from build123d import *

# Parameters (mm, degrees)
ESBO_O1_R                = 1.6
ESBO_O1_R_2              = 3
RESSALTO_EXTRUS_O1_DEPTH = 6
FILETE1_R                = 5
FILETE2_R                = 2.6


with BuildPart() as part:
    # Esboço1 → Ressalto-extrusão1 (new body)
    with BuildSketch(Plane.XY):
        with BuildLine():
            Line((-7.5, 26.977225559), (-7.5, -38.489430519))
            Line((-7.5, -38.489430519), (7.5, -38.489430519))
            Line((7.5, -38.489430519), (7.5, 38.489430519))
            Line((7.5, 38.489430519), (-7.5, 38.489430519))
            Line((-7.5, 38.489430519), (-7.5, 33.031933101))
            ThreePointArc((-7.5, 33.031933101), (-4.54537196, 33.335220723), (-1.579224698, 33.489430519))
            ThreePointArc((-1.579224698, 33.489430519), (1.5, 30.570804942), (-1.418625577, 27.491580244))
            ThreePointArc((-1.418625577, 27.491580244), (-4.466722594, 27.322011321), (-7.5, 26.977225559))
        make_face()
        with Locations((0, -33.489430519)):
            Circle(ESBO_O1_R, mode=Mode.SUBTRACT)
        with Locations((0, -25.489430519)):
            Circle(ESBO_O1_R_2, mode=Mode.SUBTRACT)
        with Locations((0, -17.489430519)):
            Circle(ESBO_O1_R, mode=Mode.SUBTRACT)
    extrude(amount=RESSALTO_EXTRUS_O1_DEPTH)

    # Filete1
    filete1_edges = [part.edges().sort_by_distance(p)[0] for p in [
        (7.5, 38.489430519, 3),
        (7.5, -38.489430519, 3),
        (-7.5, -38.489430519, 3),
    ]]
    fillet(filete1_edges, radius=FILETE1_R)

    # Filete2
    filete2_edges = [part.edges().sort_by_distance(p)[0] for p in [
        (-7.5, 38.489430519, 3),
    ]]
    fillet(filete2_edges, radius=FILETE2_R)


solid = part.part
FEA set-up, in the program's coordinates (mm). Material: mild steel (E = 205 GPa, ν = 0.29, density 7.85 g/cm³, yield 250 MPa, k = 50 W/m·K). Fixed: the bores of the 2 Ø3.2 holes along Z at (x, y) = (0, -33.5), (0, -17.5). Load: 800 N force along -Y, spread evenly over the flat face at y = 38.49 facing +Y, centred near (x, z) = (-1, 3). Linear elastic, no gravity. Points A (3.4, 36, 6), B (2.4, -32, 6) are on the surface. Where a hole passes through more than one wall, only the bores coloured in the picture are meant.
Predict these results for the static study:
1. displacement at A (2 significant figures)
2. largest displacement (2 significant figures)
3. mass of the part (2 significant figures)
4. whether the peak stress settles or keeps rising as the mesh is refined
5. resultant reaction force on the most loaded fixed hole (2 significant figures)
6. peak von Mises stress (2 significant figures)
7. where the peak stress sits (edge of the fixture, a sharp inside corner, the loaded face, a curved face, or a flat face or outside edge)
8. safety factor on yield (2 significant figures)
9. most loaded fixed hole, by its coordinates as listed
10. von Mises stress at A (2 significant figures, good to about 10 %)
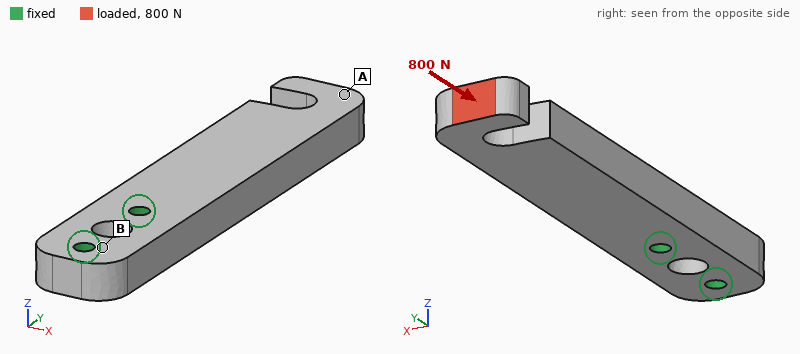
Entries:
15 µm
32 µm
49 g
settles
690 N
220 MPa
a curved face
1.2
(0, -17.5)
36 MPa
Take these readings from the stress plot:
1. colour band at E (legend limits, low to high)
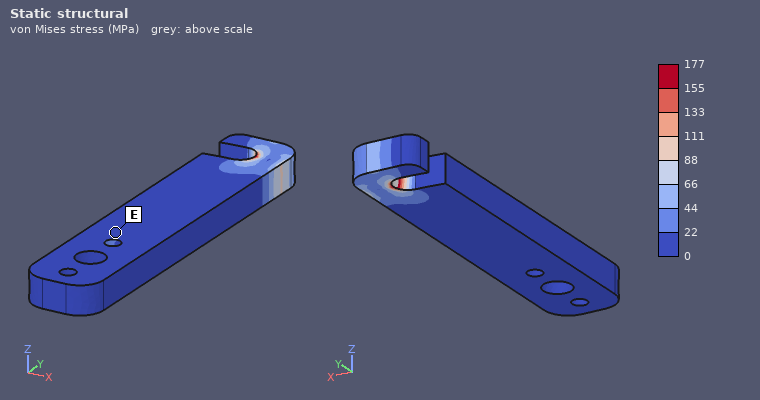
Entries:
0 to 22 MPa
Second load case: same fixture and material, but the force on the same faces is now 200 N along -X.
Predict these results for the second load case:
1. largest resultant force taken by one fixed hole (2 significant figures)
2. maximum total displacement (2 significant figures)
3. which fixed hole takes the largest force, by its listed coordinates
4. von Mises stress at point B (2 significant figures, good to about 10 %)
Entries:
600 N
57 µm
(0, -17.5)
16 MPa
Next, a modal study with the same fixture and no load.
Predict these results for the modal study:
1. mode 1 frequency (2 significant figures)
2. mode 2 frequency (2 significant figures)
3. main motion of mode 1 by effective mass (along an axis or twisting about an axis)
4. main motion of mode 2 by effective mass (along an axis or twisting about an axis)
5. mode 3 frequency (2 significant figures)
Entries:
1700 Hz
3400 Hz
along Z
along X
9000 Hz
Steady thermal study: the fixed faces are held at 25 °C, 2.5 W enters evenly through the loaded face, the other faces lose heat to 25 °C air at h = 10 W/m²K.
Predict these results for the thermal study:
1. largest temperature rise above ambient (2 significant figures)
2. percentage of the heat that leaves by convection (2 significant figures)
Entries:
41 K
15 %
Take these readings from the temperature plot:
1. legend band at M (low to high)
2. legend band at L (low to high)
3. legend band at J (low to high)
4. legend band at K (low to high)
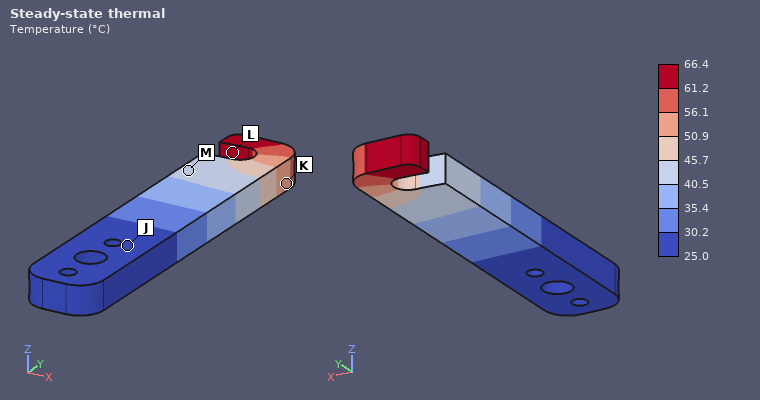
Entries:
40.5 to 45.7 °C
61.2 to 66.4 °C
25.0 to 30.2 °C
50.9 to 56.1 °C
